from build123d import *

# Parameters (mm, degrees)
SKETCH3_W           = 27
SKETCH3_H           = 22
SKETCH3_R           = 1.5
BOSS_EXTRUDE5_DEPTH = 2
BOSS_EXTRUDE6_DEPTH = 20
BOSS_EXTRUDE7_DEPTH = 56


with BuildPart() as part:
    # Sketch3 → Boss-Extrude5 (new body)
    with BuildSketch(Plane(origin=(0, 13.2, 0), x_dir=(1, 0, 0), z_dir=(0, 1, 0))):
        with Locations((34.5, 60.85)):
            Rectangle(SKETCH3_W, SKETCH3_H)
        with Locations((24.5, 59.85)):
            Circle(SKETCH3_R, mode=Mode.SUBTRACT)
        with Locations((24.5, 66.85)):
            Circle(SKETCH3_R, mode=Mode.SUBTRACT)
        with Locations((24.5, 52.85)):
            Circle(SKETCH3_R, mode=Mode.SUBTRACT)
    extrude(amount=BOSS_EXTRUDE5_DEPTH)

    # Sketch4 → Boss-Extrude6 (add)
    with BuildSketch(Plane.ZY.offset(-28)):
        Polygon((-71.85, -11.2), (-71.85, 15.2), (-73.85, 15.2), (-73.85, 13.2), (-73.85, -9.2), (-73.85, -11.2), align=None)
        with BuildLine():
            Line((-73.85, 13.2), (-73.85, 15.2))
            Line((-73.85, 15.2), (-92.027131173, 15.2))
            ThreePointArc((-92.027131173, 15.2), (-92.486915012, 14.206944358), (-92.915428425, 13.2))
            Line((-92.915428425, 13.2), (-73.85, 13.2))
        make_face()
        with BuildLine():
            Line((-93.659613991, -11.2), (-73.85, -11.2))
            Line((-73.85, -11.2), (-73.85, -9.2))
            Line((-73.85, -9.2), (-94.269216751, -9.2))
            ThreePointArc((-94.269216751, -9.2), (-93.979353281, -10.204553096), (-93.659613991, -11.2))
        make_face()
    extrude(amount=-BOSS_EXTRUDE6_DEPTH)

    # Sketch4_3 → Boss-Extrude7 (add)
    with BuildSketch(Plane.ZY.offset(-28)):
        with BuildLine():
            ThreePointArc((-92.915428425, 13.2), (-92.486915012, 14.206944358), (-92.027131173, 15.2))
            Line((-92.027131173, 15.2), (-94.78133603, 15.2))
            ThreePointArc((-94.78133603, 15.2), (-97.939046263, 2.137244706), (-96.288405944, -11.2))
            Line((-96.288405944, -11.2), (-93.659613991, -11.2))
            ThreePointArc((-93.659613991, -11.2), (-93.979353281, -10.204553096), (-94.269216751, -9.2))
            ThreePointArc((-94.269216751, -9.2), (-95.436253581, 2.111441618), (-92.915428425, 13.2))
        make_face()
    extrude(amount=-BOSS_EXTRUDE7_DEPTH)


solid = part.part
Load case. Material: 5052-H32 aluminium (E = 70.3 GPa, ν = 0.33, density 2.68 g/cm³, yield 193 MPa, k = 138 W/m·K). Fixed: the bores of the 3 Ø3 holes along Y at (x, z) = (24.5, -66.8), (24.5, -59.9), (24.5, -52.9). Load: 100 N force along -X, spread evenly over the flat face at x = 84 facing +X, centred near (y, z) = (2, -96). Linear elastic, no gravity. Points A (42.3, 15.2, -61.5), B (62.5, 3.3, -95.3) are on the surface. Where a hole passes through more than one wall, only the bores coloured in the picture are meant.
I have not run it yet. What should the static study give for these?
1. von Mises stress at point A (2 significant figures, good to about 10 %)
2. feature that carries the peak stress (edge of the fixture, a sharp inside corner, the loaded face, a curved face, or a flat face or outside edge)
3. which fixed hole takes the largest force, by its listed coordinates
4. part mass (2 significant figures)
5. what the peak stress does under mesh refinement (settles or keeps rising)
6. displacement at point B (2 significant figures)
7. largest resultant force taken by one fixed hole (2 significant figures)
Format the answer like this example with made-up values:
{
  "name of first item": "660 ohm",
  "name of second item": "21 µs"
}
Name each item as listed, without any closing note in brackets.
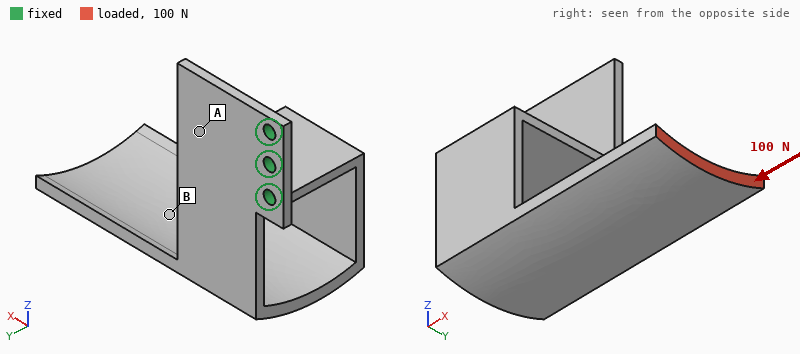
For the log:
{
  "von Mises stress at point A": "30 MPa",
  "feature that carries the peak stress": "a sharp inside corner",
  "which fixed hole takes the largest force, by its listed coordinates": "(24.5, -66.8)",
  "part mass": "20 g",
  "what the peak stress does under mesh refinement": "keeps rising",
  "displacement at point B": "0.53 mm",
  "largest resultant force taken by one fixed hole": "290 N"
}
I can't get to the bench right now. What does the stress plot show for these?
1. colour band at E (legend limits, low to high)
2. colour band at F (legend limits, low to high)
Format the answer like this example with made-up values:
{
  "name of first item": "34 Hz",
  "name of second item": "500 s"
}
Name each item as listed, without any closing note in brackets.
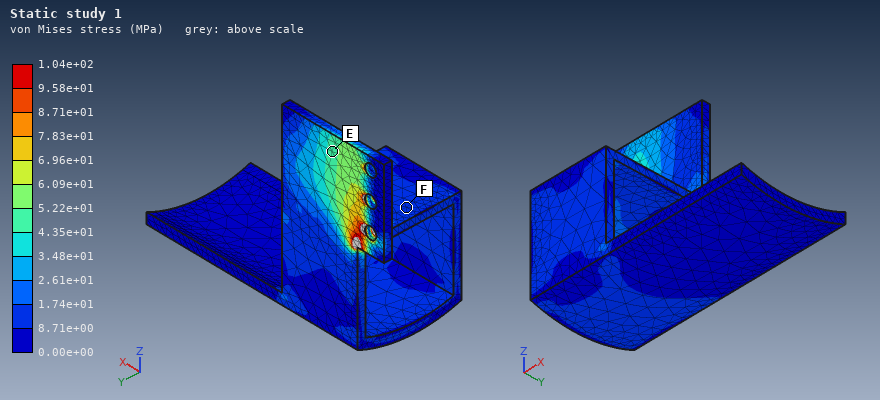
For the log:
{
  "colour band at E": "4.35e+01 to 5.22e+01 MPa",
  "colour band at F": "8.71e+00 to 1.74e+01 MPa"
}
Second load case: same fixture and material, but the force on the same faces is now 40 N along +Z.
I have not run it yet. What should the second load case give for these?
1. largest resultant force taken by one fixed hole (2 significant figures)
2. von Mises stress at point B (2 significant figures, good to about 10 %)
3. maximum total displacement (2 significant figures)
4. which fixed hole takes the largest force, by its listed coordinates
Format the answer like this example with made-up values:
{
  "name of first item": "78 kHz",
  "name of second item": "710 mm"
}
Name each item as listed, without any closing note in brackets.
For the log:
{
  "largest resultant force taken by one fixed hole": "160 N",
  "von Mises stress at point B": "8.4 MPa",
  "maximum total displacement": "0.47 mm",
  "which fixed hole takes the largest force, by its listed coordinates": "(24.5, -66.8)"
}
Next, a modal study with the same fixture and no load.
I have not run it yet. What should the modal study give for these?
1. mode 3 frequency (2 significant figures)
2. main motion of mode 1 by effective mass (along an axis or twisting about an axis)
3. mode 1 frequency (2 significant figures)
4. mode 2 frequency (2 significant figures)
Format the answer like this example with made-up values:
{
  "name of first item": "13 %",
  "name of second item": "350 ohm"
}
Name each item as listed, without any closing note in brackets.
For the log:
{
  "mode 3 frequency": "1500 Hz",
  "main motion of mode 1 by effective mass": "along Y",
  "mode 1 frequency": "300 Hz",
  "mode 2 frequency": "680 Hz"
}
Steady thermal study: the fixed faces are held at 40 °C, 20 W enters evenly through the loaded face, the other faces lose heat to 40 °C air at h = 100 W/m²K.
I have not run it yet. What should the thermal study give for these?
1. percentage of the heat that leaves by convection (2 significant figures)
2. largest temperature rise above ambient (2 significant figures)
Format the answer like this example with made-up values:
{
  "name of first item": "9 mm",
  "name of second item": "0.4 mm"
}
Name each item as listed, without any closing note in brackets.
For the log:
{
  "percentage of the heat that leaves by convection": "86 %",
  "largest temperature rise above ambient": "80 K"
}
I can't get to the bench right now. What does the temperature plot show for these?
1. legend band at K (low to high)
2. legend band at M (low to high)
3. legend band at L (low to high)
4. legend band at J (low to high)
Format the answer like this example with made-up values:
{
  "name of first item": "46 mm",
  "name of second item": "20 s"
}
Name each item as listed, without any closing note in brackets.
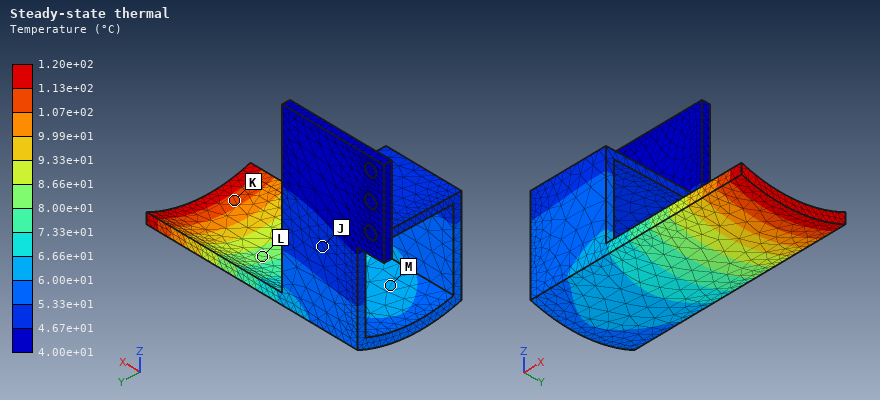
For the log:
{
  "legend band at K": "1.07e+02 to 1.13e+02 °C",
  "legend band at M": "6.00e+01 to 6.66e+01 °C",
  "legend band at L": "8.00e+01 to 8.66e+01 °C",
  "legend band at J": "4.67e+01 to 5.33e+01 °C"
}
